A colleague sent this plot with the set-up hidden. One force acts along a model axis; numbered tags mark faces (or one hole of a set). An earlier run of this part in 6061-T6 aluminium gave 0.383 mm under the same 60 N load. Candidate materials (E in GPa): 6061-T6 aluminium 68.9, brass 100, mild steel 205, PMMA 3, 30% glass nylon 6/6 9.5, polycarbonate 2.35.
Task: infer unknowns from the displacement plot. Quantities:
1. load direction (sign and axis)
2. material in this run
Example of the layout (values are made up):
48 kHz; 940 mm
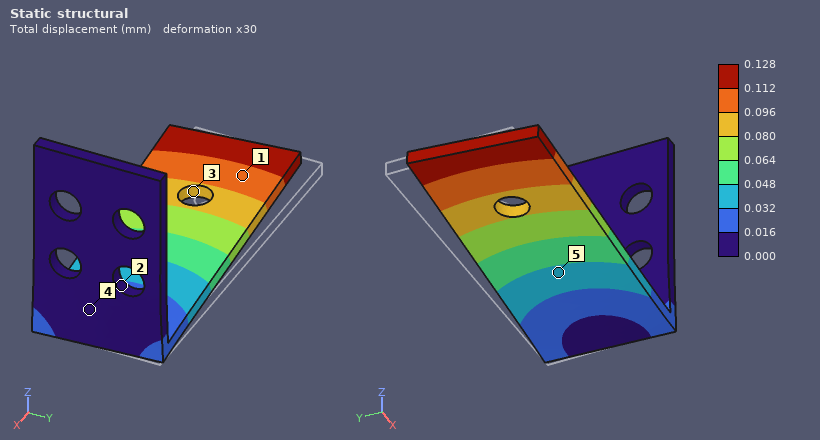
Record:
-Y; mild steel
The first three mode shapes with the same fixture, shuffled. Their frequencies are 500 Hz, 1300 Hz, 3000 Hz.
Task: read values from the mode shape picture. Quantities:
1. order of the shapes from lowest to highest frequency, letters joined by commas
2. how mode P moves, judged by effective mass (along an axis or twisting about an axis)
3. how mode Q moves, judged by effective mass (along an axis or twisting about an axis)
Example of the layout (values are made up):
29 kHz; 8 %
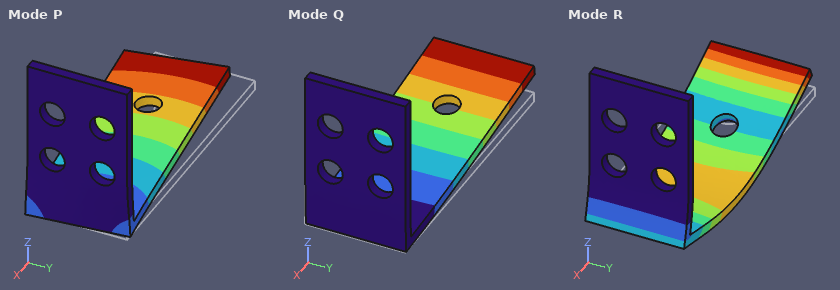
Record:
Q, P, R; along Y; along Z
